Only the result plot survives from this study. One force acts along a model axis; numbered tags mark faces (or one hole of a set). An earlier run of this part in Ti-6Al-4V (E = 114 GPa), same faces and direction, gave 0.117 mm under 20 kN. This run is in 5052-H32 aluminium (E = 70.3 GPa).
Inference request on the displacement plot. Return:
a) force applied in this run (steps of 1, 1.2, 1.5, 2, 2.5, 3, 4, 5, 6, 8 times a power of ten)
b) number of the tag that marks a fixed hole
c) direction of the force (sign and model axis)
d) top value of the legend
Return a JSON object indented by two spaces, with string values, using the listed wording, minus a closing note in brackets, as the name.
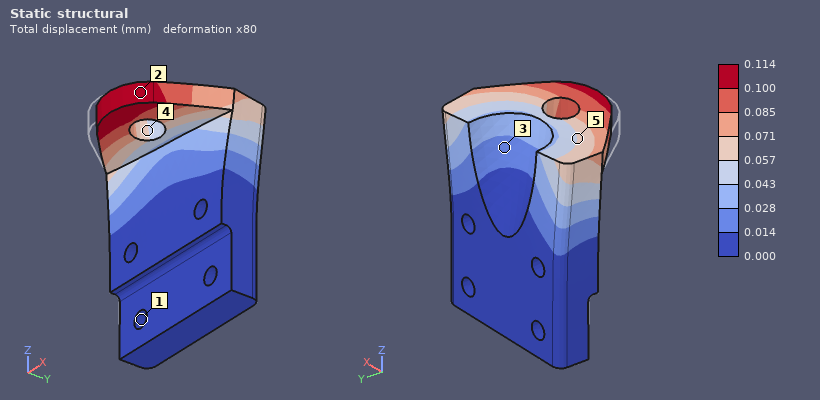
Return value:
{
  "force applied in this run": "12 kN",
  "number of the tag that marks a fixed hole": "1",
  "direction of the force": "+X",
  "top value of the legend": "0.114 mm"
}
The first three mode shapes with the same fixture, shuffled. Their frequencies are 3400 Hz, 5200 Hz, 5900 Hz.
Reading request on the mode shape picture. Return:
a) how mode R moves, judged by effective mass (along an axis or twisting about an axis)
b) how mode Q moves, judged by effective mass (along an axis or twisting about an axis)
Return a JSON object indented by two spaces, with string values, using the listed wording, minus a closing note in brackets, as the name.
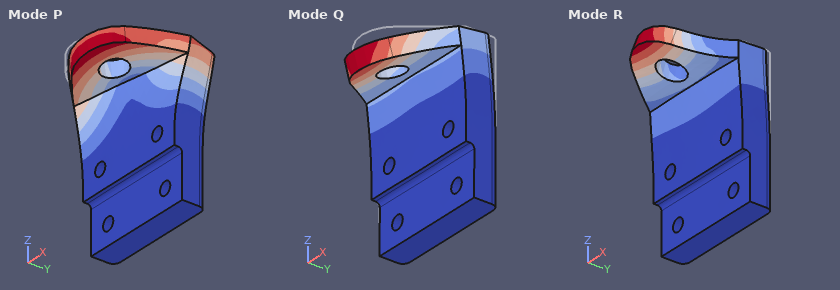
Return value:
{
  "how mode R moves, judged by effective mass": "along Y",
  "how mode Q moves, judged by effective mass": "along Y"
}
